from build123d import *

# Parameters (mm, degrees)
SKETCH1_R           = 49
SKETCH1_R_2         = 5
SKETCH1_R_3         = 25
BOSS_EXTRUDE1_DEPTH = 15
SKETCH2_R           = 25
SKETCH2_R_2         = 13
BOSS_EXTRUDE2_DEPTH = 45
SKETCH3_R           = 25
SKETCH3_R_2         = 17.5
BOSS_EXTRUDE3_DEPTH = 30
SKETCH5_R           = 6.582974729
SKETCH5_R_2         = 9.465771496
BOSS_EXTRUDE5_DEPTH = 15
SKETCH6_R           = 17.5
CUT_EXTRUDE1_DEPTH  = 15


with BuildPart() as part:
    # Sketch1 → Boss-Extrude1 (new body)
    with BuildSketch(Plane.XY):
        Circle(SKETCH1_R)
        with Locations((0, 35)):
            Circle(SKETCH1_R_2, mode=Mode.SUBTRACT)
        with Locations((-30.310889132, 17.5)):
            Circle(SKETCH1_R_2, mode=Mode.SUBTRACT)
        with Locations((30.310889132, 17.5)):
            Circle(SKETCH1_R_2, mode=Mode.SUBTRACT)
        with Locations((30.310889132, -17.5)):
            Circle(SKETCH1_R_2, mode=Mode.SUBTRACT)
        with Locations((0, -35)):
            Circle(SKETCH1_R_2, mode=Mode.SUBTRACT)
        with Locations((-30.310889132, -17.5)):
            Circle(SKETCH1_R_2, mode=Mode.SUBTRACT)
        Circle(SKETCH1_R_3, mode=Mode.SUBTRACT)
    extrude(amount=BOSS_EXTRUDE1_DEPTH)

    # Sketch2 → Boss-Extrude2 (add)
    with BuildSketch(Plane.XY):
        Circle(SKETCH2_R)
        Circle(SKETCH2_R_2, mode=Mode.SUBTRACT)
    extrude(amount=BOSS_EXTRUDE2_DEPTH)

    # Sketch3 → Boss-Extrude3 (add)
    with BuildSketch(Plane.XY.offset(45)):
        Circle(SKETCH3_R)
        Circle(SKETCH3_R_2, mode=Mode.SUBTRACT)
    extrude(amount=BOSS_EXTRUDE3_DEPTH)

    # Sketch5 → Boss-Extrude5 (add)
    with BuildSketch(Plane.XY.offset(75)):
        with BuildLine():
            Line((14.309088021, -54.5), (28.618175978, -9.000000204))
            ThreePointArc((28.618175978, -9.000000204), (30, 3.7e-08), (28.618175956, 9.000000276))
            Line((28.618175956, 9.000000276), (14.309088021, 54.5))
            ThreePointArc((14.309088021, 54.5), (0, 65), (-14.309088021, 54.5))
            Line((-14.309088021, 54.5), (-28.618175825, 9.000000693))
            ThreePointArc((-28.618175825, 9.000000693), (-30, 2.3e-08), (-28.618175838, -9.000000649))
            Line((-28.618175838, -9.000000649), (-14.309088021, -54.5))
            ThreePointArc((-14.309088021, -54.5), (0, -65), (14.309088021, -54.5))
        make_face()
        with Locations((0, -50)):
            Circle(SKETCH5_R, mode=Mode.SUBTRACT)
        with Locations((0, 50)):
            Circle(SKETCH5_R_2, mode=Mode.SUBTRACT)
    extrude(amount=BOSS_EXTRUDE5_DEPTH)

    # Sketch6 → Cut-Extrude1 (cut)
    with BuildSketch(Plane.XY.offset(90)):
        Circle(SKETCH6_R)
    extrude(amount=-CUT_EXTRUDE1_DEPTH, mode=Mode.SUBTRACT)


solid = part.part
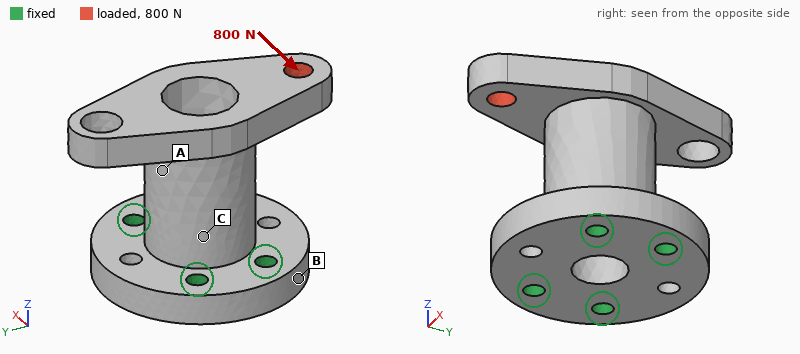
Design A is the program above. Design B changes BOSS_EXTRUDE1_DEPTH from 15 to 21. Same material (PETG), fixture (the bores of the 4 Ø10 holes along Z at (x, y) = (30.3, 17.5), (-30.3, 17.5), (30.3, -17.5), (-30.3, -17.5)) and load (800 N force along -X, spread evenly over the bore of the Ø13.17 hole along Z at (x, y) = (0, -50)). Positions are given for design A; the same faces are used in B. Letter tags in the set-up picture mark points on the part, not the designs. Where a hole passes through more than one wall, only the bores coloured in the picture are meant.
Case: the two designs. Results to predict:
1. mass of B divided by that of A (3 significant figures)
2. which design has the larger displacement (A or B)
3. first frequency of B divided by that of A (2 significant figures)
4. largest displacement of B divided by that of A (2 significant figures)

1.13
A
1.2
0.88
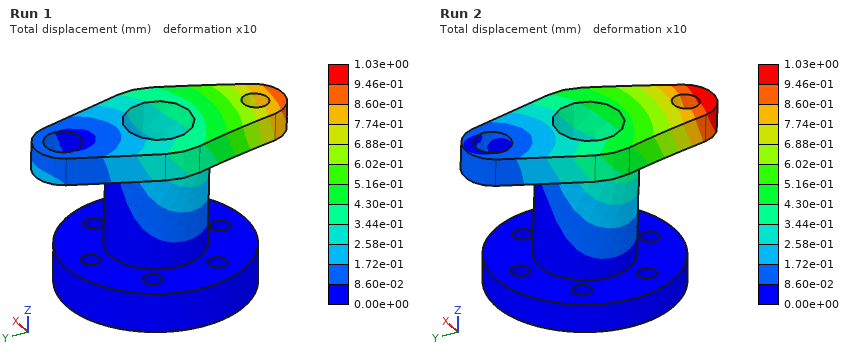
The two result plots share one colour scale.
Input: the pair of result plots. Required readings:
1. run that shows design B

Run 1
